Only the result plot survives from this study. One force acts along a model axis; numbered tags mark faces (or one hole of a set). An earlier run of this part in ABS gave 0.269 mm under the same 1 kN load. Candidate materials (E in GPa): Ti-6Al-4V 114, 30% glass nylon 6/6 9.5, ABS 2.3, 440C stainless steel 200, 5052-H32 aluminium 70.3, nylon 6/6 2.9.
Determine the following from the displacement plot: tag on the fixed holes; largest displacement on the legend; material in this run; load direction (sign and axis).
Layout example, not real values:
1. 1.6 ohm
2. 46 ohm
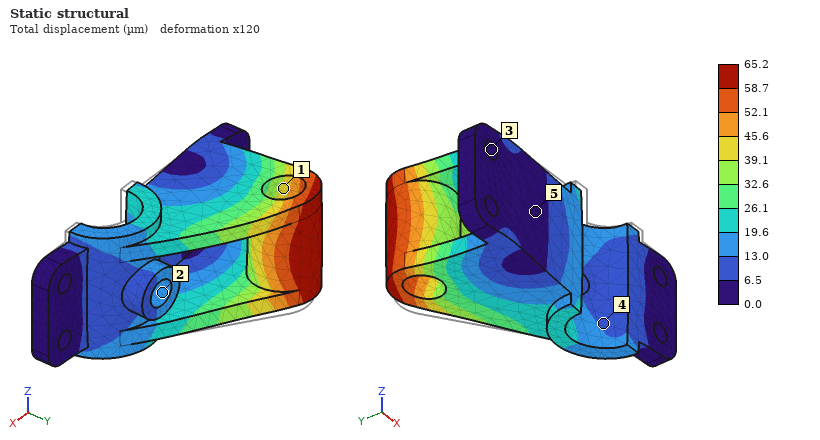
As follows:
1. 3
2. 65.2 µm
3. 30% glass nylon 6/6
4. -X
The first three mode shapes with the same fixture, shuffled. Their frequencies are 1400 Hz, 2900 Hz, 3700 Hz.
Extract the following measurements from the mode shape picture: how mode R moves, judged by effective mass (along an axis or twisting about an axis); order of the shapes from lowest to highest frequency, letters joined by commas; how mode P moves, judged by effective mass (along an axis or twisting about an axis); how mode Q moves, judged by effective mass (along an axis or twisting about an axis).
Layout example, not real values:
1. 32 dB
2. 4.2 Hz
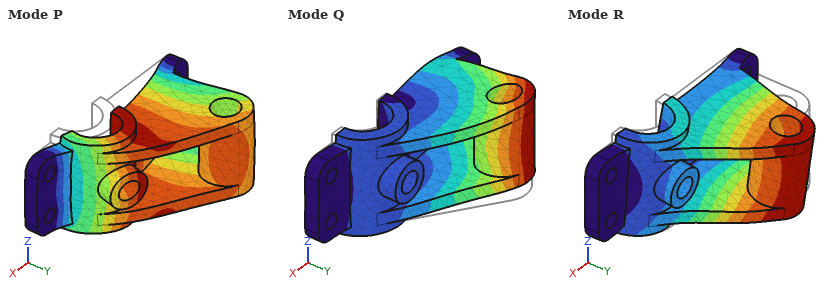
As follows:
1. along Z
2. R, P, Q
3. along Y
4. along X
